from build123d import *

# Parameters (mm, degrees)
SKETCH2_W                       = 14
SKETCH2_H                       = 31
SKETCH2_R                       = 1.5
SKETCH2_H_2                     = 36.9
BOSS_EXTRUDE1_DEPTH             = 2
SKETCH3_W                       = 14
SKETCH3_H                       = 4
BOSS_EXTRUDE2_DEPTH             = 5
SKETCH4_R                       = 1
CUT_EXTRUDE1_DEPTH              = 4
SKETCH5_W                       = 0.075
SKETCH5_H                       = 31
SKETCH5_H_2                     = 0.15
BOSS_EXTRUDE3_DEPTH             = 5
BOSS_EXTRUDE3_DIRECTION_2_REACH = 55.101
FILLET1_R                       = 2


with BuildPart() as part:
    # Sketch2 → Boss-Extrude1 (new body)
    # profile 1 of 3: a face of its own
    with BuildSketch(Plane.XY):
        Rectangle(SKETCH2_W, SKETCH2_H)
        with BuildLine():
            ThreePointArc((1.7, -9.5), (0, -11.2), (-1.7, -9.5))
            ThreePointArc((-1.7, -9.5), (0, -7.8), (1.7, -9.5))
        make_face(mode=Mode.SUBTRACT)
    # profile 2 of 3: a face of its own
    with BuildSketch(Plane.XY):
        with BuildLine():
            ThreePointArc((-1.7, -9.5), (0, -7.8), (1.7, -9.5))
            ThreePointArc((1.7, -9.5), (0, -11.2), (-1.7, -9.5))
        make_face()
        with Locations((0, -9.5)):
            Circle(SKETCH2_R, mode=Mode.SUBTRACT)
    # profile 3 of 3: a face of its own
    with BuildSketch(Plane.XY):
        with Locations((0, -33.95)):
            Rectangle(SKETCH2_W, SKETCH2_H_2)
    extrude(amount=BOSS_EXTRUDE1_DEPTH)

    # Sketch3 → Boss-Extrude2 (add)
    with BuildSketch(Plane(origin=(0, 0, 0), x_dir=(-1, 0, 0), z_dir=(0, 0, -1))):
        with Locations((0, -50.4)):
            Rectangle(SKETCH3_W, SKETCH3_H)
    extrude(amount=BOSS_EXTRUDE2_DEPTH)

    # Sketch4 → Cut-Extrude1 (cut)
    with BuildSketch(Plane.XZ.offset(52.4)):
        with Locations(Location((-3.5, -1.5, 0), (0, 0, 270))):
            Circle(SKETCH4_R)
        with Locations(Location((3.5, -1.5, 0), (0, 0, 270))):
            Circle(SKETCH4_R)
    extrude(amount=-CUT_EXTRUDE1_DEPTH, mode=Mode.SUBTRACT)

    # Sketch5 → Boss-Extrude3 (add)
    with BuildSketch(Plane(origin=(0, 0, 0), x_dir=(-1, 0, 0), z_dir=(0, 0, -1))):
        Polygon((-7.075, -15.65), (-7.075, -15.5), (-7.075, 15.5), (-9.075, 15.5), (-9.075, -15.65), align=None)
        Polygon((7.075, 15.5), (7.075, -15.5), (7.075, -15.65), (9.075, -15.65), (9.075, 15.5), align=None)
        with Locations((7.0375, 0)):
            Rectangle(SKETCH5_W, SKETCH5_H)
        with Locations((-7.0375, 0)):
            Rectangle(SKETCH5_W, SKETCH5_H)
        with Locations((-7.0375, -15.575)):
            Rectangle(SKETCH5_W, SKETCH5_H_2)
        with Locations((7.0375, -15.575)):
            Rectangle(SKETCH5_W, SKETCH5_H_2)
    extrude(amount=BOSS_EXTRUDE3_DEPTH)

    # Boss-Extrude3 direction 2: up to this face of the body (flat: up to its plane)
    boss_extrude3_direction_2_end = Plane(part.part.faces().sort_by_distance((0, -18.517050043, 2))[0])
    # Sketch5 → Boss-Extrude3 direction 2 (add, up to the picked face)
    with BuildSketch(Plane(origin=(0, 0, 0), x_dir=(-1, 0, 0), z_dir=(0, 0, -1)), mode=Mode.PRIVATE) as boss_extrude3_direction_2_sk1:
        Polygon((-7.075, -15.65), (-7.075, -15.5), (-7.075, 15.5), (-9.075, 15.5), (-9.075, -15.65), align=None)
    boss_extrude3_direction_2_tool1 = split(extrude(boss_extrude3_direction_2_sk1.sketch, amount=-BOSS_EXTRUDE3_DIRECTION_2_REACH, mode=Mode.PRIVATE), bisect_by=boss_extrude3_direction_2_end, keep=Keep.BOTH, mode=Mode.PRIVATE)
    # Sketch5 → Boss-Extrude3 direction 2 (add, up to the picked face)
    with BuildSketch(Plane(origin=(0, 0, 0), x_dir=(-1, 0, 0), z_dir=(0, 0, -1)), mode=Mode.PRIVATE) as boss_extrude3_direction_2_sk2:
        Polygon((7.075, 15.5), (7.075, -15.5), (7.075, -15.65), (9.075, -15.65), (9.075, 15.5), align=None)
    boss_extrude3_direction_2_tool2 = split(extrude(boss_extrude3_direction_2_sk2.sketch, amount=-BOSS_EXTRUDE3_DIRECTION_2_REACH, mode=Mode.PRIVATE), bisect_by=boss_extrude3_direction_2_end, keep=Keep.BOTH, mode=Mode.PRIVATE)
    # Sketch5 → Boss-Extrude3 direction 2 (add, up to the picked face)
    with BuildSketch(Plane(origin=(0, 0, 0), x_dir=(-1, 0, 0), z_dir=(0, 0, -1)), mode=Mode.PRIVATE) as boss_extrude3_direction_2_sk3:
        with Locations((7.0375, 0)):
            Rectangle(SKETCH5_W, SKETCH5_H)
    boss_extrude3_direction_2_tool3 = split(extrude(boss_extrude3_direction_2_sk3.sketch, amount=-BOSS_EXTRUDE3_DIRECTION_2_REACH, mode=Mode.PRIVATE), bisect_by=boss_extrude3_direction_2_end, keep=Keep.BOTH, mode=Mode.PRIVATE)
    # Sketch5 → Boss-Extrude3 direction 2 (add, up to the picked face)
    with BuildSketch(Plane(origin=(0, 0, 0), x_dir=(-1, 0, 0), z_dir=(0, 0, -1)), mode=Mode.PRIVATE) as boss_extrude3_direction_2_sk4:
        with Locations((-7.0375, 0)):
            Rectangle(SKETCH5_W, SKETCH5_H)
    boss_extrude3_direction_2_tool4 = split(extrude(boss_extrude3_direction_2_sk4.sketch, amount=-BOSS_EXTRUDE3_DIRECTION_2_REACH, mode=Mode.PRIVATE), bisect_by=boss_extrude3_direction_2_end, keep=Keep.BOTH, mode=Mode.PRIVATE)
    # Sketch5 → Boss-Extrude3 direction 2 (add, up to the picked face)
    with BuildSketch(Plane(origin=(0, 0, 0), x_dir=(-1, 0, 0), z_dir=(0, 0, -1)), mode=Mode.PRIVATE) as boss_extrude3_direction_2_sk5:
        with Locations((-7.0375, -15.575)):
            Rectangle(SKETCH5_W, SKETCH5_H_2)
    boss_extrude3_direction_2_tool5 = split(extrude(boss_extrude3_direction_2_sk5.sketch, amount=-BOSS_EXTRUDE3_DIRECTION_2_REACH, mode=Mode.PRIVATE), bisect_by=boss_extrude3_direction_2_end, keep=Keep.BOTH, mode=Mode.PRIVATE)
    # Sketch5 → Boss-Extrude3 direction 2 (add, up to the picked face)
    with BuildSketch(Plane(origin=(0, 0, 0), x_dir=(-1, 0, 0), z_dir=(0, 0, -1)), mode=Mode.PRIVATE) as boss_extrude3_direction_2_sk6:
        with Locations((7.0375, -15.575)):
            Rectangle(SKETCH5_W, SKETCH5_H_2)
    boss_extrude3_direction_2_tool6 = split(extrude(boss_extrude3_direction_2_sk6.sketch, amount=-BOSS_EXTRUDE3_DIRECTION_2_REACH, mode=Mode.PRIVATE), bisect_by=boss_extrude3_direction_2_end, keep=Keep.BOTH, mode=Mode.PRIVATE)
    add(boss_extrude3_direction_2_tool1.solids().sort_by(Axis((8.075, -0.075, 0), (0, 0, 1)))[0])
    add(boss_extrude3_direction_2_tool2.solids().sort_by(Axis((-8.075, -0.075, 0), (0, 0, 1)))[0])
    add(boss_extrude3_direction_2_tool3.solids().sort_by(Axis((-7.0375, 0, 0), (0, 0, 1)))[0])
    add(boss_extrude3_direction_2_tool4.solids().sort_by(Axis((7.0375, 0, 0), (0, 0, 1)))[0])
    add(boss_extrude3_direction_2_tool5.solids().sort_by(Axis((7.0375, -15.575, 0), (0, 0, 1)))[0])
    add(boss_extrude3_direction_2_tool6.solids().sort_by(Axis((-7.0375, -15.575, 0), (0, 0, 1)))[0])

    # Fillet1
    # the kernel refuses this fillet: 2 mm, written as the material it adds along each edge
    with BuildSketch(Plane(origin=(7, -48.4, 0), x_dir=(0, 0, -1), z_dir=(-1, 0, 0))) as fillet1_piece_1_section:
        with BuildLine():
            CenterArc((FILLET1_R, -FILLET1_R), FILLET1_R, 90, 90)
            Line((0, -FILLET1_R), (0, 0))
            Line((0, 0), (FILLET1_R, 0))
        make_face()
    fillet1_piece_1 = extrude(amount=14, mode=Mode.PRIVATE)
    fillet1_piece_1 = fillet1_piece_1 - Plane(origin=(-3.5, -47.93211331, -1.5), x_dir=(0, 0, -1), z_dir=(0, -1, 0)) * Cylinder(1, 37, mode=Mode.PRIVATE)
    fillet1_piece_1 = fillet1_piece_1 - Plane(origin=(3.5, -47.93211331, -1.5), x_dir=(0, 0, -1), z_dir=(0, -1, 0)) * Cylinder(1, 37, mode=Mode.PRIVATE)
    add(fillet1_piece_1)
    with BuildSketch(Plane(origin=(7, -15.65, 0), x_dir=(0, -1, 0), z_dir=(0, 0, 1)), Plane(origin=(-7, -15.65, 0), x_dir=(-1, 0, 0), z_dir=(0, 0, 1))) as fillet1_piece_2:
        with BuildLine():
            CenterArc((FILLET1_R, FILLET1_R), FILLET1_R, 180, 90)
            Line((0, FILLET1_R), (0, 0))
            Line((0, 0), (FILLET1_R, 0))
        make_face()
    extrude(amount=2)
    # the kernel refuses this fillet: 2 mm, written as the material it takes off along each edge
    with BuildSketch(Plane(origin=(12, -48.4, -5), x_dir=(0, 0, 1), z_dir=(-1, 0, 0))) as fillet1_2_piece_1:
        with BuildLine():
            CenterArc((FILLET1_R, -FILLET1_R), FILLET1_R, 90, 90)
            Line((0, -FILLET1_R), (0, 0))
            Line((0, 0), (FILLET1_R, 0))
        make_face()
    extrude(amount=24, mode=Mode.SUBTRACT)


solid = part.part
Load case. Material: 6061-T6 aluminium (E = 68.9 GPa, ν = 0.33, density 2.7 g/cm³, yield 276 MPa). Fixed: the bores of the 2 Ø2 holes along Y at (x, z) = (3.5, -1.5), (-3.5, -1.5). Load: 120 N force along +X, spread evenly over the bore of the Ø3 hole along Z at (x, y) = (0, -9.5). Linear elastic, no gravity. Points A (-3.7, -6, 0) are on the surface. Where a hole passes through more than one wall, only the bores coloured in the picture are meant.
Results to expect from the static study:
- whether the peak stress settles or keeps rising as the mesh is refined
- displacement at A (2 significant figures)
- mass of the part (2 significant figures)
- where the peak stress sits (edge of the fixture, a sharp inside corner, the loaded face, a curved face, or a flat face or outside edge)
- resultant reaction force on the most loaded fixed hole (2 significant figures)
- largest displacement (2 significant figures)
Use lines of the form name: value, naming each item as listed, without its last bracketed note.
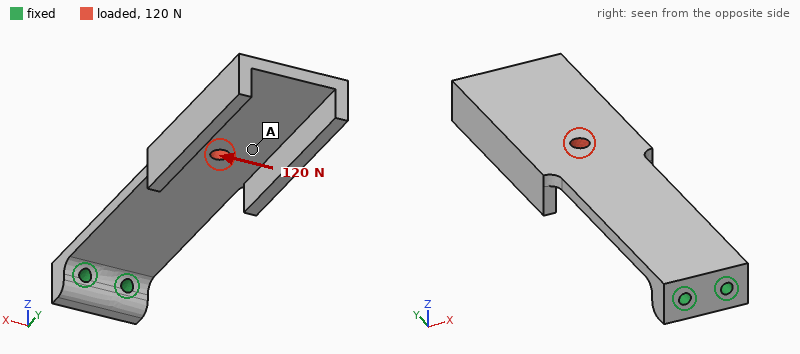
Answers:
whether the peak stress settles or keeps rising as the mesh is refined: keeps rising
displacement at A: 0.12 mm
mass of the part: 8.2 g
where the peak stress sits: edge of the fixture
resultant reaction force on the most loaded fixed hole: 490 N
largest displacement: 0.20 mm
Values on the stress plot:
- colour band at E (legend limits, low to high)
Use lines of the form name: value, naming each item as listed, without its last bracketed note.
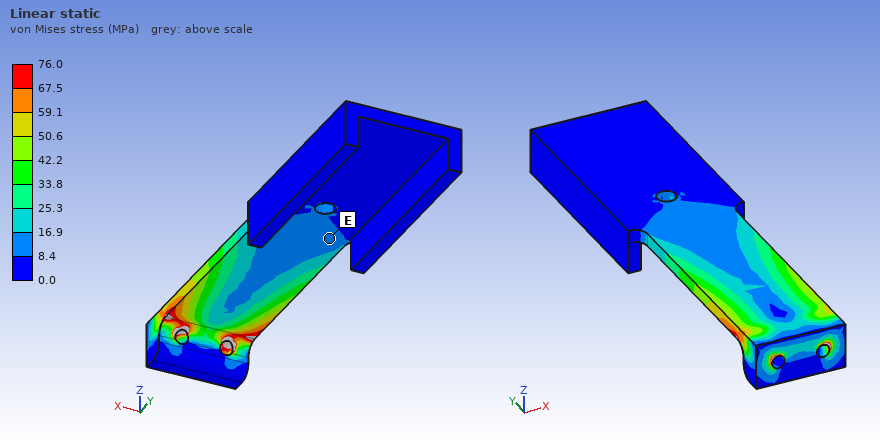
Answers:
colour band at E: 8.4 to 16.9 MPa
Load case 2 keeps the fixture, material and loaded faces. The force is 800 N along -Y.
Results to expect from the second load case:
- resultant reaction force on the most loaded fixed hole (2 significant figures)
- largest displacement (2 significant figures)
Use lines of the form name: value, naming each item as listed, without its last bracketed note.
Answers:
resultant reaction force on the most loaded fixed hole: 400 N
largest displacement: 75 µm
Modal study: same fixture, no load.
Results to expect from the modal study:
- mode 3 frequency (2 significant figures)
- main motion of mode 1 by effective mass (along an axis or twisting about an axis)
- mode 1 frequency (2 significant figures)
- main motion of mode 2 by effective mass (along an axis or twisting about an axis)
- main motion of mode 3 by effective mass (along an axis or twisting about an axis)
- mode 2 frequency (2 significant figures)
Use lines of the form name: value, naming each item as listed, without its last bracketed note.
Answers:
mode 3 frequency: 1900 Hz
main motion of mode 1 by effective mass: along Z
mode 1 frequency: 290 Hz
main motion of mode 2 by effective mass: along X
main motion of mode 3 by effective mass: along X
mode 2 frequency: 1500 Hz
